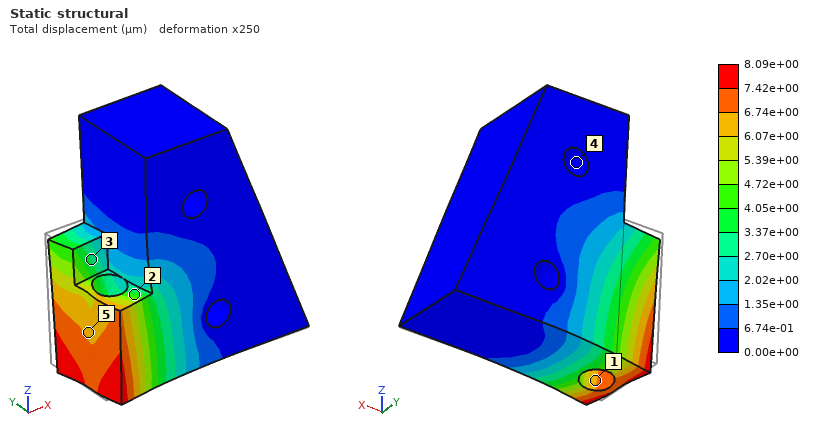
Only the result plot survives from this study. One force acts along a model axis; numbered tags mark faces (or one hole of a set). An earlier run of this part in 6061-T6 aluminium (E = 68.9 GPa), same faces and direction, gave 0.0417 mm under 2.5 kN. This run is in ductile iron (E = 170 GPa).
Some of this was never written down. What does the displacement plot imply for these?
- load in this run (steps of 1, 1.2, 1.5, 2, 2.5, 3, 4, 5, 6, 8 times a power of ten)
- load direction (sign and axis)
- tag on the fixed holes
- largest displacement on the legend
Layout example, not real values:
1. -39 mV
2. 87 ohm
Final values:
1. 1.2 kN
2. -Y
3. 4
4. 8.09e+00 µm
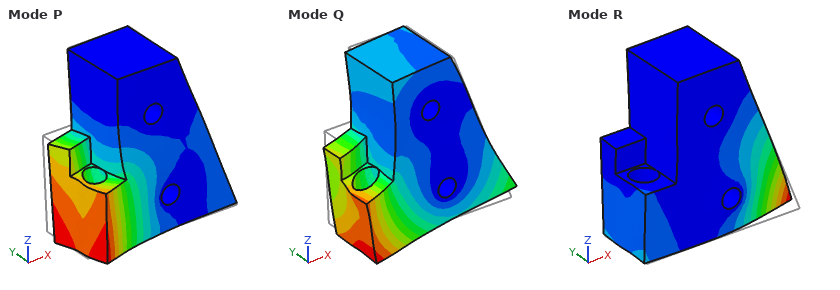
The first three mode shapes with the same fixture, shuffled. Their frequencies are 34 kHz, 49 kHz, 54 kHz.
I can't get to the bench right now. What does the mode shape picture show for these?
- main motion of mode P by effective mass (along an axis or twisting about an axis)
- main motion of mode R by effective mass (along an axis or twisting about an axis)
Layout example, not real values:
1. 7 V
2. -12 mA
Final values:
1. along Y
2. along Y
